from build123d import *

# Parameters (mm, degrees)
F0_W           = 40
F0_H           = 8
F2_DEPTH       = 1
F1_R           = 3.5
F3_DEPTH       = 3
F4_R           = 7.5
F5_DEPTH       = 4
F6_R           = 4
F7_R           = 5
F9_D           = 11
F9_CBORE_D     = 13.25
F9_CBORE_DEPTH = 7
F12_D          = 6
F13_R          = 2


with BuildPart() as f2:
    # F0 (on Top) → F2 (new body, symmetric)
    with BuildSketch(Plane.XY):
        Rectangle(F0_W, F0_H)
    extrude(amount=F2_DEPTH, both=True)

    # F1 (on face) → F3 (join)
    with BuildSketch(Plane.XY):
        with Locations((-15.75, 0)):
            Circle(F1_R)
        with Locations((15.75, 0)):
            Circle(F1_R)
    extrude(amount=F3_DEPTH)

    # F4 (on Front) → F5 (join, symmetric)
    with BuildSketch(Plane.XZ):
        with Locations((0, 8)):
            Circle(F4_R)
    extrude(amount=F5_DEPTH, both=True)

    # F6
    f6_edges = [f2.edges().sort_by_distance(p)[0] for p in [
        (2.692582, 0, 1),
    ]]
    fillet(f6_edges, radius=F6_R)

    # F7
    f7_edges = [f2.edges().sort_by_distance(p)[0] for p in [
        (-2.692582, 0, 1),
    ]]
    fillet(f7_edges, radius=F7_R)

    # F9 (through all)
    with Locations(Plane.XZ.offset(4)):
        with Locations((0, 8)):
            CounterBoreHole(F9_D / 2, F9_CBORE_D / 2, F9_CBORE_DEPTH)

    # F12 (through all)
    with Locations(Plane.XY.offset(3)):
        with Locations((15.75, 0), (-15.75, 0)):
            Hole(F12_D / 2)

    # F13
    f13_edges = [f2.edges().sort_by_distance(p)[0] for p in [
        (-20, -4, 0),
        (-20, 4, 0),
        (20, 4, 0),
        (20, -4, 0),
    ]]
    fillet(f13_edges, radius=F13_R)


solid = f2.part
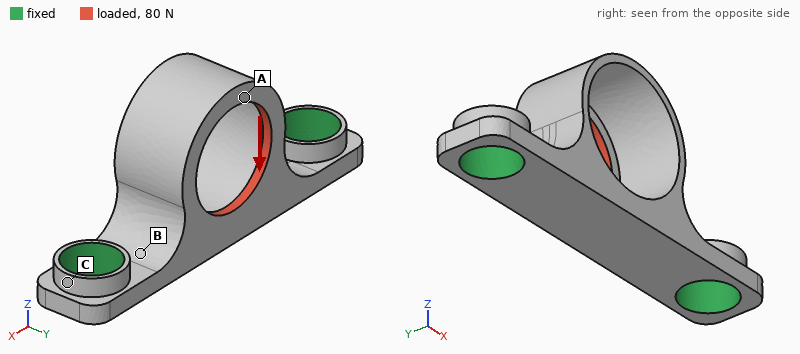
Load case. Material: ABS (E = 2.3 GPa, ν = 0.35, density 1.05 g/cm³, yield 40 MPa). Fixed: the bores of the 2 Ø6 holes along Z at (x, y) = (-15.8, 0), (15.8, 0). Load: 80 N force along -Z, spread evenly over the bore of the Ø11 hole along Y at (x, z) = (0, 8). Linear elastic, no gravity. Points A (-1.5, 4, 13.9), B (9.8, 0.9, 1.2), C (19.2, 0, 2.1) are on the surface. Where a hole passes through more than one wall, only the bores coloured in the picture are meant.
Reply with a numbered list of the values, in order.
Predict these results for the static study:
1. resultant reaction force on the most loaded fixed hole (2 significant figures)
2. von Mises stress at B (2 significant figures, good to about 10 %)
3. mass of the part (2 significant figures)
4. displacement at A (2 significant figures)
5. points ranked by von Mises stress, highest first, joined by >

1. 52 N
2. 13 MPa
3. 1.1 g
4. 0.41 mm
5. B > A > C
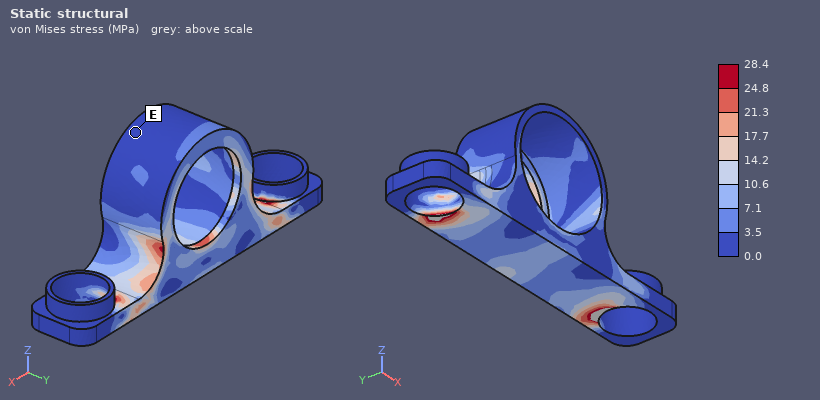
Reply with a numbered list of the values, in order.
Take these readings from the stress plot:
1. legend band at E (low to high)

1. 0.0 to 3.5 MPa
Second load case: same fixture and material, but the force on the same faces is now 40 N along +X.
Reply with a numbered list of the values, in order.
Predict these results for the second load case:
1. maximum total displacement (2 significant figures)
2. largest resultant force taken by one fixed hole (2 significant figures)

1. 0.23 mm
2. 25 N
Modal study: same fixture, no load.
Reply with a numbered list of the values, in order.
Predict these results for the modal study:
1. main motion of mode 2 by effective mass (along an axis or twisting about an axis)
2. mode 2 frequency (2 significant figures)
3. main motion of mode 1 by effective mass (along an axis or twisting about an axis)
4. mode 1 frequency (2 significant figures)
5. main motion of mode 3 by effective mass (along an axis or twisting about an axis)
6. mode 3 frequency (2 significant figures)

1. along X
2. 3500 Hz
3. along Y
4. 2700 Hz
5. along Z
6. 4300 Hz
